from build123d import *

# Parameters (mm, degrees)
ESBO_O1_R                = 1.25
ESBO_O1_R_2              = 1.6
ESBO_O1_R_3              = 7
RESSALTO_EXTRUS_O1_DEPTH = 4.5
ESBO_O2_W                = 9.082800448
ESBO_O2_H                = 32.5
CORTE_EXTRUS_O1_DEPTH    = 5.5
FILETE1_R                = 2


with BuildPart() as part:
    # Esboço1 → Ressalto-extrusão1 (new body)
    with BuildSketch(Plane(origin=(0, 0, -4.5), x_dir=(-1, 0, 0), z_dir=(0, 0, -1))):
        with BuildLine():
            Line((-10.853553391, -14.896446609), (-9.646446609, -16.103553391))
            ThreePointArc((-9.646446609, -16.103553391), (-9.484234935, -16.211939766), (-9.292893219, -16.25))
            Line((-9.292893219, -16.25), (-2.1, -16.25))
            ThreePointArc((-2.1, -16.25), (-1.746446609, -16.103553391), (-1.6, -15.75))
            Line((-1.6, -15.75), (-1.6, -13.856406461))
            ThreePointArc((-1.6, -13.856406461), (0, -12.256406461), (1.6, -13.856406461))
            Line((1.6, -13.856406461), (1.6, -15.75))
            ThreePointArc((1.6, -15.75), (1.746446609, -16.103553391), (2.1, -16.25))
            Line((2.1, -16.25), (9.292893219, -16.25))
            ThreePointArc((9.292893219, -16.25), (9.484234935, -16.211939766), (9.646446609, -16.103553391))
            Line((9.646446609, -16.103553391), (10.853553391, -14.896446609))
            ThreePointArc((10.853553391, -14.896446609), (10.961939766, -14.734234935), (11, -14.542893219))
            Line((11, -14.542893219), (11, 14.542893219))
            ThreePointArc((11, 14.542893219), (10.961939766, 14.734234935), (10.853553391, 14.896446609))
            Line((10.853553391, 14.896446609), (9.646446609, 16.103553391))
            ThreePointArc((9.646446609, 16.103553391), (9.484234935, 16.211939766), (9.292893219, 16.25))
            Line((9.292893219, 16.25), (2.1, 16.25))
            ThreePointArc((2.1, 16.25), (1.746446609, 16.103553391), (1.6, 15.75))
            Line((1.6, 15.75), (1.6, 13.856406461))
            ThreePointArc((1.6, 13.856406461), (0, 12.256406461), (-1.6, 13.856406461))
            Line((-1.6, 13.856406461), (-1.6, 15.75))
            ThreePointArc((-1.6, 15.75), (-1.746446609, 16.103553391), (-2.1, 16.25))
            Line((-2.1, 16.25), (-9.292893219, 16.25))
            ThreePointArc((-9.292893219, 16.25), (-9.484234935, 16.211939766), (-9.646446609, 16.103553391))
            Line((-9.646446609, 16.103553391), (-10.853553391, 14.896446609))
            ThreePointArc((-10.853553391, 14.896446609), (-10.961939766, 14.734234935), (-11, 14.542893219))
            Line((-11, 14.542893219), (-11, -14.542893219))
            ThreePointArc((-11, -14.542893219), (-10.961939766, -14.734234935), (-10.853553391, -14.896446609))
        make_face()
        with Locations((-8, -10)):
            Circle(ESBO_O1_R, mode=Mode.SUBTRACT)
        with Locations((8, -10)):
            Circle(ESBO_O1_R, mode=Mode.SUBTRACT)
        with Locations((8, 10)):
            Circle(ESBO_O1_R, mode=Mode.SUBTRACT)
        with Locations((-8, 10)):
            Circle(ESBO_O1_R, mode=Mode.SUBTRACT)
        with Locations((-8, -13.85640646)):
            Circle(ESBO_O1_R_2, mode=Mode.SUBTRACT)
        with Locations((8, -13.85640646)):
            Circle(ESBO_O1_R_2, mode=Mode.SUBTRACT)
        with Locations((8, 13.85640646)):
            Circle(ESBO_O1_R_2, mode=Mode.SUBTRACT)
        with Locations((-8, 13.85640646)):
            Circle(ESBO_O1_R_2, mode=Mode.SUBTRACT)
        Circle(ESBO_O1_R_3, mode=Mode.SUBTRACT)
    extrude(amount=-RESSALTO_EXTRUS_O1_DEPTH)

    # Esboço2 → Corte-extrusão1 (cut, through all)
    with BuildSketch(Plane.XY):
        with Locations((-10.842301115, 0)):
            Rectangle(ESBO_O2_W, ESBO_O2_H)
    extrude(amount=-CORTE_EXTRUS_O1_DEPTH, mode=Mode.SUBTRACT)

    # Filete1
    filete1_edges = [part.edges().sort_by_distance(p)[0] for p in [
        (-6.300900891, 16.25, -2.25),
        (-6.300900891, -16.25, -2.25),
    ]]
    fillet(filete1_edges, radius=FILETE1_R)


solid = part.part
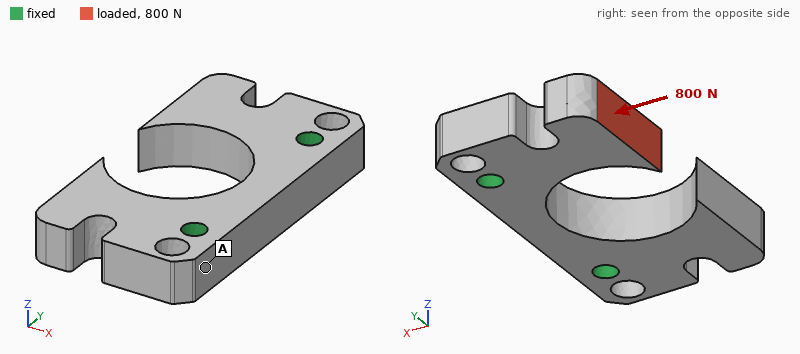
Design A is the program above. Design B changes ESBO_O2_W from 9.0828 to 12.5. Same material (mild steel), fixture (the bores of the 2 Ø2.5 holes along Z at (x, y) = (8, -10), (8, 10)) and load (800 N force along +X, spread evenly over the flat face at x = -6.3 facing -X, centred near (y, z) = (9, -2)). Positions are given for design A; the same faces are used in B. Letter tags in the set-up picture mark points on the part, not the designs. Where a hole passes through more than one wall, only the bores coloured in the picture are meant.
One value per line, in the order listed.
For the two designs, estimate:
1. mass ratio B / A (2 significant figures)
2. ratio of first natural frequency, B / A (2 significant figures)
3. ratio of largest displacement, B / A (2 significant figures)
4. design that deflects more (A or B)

0.89
1.4
0.19
A
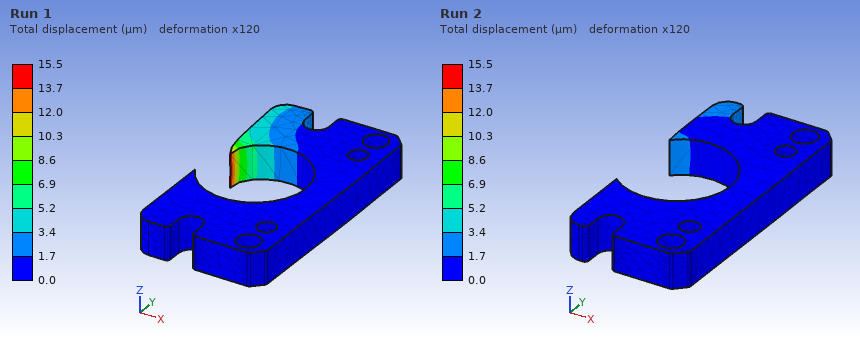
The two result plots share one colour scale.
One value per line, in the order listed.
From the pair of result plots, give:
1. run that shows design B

Run 2
